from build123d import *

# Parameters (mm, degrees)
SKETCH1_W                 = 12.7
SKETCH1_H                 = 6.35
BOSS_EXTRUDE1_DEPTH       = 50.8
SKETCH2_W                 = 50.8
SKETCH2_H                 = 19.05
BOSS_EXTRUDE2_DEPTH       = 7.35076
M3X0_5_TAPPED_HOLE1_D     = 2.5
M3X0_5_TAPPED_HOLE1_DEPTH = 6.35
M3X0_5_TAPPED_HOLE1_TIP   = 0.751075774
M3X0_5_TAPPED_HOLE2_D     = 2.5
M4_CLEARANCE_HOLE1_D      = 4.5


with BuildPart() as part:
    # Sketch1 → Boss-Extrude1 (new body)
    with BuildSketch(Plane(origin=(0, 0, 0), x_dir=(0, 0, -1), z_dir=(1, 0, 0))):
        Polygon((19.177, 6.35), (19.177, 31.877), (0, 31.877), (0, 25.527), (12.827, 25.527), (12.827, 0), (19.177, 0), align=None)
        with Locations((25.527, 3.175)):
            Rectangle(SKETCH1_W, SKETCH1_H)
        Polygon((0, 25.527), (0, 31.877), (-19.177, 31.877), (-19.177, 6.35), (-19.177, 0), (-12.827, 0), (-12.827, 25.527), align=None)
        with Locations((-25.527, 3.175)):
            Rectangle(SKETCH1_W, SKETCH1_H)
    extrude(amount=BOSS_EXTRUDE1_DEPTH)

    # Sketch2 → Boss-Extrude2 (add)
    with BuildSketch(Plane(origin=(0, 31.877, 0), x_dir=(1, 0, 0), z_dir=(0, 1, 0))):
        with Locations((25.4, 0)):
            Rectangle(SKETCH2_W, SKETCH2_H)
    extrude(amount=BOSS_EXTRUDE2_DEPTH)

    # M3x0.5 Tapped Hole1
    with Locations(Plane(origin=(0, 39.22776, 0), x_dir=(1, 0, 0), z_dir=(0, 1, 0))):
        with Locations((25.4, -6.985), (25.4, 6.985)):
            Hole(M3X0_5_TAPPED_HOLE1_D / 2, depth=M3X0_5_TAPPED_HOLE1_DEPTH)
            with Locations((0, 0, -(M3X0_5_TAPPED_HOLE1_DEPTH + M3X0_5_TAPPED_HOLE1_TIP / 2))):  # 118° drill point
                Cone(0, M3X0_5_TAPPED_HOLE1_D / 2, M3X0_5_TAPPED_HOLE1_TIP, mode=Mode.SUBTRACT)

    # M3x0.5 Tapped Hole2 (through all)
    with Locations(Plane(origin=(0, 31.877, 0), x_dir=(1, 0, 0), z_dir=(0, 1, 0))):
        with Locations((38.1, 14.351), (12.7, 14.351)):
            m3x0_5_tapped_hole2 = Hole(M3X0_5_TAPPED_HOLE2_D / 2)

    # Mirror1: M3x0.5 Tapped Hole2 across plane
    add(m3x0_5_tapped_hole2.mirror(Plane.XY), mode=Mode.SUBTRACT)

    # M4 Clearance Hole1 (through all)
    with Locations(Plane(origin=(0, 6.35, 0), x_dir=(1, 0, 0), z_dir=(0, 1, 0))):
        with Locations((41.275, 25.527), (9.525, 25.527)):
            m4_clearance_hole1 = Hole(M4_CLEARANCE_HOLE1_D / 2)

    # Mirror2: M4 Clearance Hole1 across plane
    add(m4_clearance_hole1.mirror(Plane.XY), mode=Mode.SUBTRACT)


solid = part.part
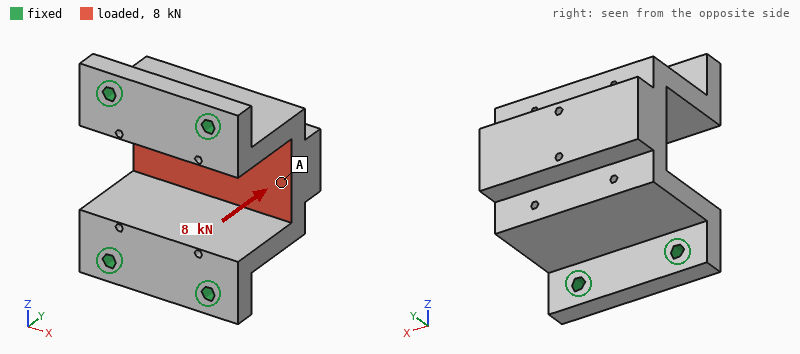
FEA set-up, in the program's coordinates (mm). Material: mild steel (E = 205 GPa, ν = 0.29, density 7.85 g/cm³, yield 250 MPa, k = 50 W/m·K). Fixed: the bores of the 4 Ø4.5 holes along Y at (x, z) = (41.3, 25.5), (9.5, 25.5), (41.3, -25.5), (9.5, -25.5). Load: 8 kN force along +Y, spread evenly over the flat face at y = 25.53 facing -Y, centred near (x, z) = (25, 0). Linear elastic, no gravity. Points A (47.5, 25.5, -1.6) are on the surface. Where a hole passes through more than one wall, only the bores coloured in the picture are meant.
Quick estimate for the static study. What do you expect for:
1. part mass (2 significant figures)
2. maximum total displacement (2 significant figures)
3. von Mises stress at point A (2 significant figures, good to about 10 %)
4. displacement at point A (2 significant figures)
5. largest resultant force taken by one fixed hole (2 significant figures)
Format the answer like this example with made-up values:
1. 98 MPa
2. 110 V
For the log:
1. 340 g
2. 8.7 µm
3. 12 MPa
4. 8.5 µm
5. 2.1 kN
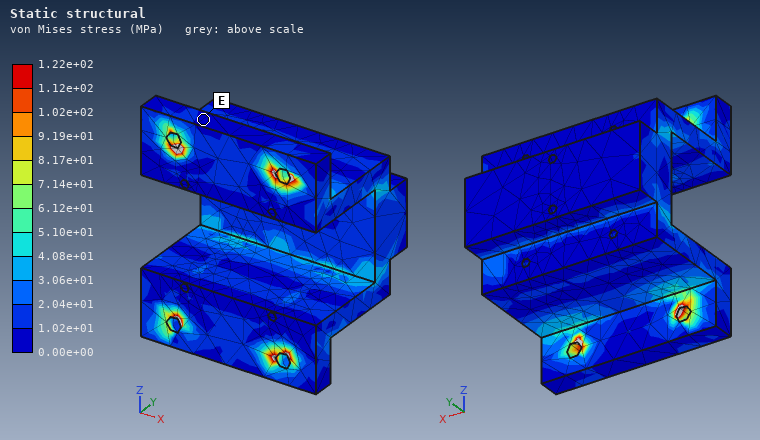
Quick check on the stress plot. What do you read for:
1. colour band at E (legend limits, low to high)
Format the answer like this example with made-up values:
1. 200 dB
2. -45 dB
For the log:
1. 0.00e+00 to 1.02e+01 MPa
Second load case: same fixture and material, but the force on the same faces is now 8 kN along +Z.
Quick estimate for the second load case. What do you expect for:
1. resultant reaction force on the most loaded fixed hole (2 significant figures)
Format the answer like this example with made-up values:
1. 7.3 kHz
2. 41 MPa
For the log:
1. 2.5 kN
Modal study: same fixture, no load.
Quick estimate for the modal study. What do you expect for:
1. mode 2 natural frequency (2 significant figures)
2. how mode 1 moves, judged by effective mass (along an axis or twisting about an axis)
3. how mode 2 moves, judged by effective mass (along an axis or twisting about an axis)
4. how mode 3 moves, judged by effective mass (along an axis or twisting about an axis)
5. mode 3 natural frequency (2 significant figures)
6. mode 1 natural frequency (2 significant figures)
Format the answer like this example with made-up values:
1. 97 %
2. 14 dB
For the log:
1. 6600 Hz
2. along Z
3. along X
4. twisting about Y
5. 8400 Hz
6. 5000 Hz
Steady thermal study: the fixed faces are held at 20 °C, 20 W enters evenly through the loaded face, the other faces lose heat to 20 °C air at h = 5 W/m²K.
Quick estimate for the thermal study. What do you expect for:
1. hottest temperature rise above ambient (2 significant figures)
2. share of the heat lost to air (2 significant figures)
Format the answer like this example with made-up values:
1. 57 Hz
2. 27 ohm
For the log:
1. 26 K
2. 4.6 %
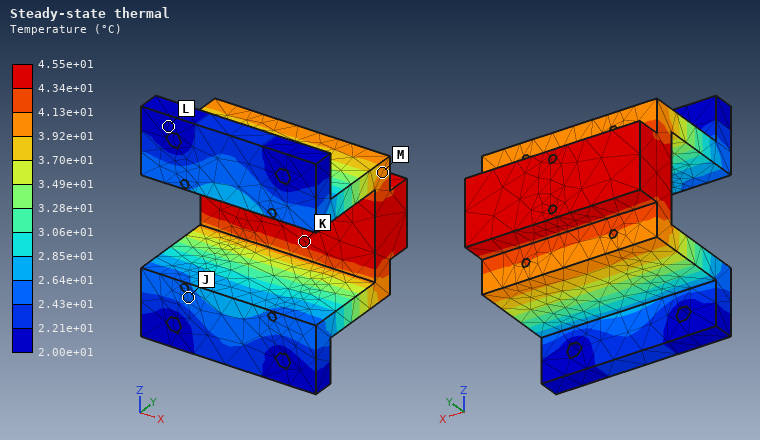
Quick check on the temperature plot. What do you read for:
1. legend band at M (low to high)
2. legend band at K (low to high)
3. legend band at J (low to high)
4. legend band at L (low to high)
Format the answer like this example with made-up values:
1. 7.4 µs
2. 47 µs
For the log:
1. 3.92e+01 to 4.13e+01 °C
2. 4.34e+01 to 4.55e+01 °C
3. 2.43e+01 to 2.64e+01 °C
4. 2.00e+01 to 2.21e+01 °C
